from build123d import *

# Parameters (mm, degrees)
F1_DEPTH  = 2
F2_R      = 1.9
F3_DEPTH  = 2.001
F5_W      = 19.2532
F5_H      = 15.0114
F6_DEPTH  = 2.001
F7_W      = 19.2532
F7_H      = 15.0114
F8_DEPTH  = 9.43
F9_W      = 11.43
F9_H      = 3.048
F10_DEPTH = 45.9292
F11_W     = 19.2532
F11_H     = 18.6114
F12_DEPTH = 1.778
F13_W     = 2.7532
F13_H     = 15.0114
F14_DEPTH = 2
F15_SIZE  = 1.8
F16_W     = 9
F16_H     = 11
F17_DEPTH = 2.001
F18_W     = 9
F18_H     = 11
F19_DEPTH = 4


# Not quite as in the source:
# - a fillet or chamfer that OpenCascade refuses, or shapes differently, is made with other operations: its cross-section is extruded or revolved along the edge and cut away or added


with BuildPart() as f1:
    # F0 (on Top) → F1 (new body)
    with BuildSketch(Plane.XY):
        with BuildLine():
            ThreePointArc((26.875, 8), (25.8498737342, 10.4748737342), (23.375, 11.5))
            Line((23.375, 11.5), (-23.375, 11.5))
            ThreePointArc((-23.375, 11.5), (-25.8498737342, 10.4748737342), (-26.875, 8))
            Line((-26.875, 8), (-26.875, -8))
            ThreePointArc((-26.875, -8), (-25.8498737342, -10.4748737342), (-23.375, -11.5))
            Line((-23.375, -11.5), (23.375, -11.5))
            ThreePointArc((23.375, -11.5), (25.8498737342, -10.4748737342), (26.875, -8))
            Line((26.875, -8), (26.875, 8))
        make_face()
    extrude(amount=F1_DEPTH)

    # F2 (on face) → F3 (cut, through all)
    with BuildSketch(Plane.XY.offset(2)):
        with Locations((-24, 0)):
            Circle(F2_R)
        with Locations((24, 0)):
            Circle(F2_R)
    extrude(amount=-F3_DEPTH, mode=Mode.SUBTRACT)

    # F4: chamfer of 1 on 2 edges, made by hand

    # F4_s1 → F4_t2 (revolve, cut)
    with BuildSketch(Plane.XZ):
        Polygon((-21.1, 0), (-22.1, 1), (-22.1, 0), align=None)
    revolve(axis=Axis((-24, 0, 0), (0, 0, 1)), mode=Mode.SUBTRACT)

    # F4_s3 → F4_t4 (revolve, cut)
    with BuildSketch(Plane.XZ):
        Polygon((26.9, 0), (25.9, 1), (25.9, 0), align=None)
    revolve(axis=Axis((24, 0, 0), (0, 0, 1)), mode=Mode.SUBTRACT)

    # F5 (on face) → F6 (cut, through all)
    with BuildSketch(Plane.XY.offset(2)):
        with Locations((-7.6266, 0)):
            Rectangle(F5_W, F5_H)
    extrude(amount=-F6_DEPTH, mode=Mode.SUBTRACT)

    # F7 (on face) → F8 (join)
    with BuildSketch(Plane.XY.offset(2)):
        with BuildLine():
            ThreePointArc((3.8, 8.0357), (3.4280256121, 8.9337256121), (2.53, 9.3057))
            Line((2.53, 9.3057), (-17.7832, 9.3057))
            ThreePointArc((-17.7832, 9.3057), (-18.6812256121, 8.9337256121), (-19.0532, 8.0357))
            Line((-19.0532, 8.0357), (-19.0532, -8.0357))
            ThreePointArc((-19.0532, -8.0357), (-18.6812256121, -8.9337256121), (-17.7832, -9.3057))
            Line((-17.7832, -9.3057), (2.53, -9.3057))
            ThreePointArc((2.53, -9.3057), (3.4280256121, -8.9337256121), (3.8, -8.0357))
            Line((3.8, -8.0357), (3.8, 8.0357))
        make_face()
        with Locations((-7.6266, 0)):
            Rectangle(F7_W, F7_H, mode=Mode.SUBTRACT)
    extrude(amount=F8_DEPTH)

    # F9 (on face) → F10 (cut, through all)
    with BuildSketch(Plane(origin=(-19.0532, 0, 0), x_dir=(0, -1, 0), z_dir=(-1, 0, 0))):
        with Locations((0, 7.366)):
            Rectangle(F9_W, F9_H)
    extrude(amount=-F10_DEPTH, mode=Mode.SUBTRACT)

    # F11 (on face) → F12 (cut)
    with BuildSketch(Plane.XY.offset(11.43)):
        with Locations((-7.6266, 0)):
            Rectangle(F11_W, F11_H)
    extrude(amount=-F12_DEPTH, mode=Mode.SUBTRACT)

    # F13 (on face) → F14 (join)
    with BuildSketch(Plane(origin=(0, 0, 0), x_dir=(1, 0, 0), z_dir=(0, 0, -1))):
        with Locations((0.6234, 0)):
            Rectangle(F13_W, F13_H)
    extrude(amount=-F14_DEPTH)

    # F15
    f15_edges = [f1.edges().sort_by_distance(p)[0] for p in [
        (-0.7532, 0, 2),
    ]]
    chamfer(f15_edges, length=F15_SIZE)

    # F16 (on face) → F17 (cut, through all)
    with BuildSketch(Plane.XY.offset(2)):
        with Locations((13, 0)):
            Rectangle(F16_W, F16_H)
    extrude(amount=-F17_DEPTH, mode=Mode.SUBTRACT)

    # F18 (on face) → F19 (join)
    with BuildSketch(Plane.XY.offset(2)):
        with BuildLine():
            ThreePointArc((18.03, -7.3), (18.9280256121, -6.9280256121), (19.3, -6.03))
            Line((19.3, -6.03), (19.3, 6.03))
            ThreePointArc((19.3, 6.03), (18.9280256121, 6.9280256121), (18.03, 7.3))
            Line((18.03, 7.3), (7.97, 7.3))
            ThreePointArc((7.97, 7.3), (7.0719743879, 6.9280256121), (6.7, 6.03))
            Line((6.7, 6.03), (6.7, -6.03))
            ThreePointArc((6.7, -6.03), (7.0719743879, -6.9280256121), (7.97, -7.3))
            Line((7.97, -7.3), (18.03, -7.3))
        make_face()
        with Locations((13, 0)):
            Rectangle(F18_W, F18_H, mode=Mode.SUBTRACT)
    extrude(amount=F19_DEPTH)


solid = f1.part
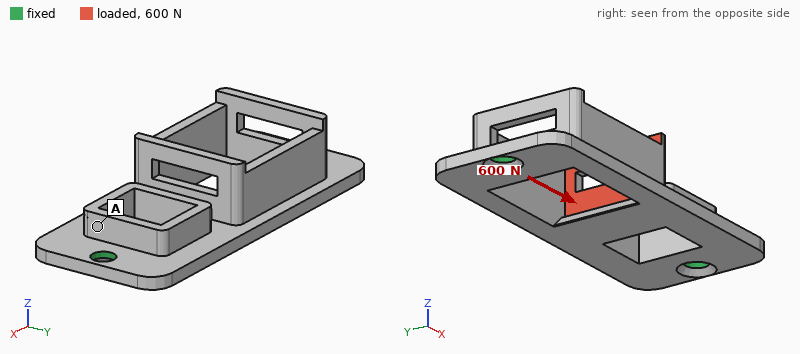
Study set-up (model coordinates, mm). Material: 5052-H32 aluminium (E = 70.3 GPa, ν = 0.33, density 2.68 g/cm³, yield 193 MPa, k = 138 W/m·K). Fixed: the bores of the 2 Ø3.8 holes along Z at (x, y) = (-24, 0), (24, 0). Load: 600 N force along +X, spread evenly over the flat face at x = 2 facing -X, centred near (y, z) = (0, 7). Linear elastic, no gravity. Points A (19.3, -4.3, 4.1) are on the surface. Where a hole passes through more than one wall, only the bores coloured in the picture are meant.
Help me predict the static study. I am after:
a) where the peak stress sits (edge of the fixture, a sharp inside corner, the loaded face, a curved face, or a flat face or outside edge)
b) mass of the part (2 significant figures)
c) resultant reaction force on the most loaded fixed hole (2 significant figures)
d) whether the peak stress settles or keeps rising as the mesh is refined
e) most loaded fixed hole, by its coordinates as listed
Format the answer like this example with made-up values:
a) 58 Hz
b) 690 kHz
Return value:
a) edge of the fixture
b) 8.1 g
c) 330 N
d) keeps rising
e) (24, 0)
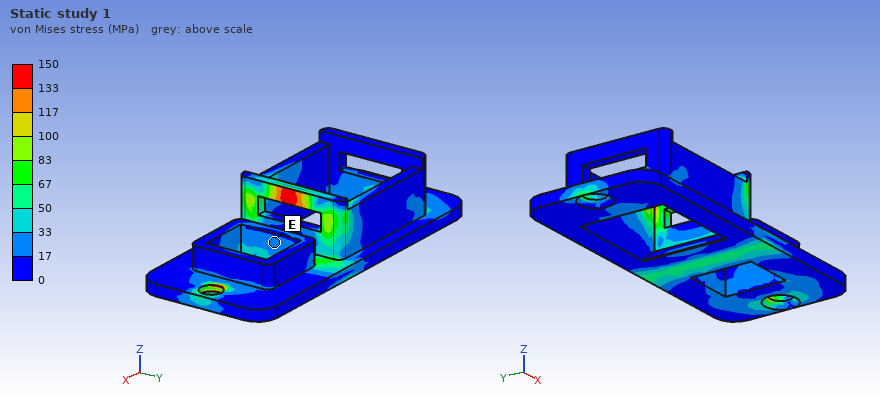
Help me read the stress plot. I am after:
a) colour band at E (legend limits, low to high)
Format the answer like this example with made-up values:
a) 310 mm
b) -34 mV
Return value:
a) 17 to 33 MPa
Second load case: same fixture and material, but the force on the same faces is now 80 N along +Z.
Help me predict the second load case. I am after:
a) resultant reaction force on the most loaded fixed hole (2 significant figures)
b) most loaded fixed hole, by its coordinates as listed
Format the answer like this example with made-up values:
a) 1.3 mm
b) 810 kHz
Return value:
a) 47 N
b) (24, 0)
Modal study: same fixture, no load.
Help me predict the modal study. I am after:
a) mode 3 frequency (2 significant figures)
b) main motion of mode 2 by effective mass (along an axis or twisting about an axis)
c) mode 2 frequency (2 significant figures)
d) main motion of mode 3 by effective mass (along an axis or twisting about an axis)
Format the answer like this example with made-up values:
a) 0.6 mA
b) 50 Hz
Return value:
a) 9100 Hz
b) along Z
c) 4000 Hz
d) along Y
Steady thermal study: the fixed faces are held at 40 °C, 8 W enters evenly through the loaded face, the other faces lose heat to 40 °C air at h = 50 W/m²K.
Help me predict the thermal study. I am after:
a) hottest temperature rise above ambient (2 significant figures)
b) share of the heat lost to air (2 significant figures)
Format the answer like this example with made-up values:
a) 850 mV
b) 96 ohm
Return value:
a) 30 K
b) 23 %
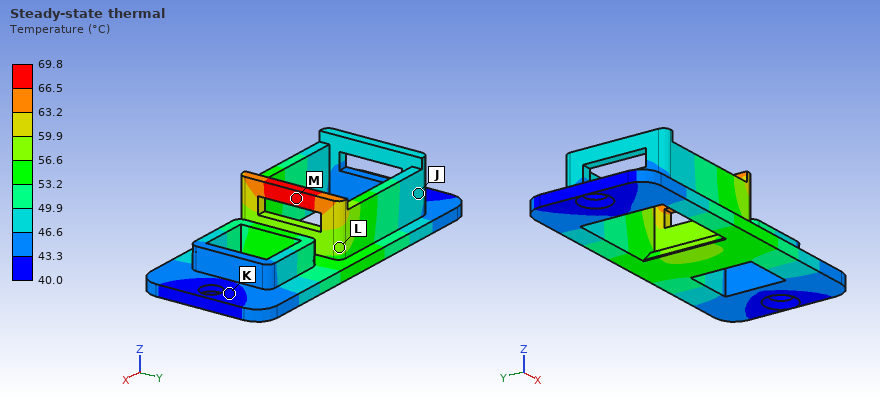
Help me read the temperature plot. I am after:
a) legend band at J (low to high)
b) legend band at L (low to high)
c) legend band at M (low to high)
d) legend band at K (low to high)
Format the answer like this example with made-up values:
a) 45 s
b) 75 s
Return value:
a) 46.6 to 49.9 °C
b) 56.6 to 59.9 °C
c) 66.5 to 69.8 °C
d) 40.0 to 43.3 °C
